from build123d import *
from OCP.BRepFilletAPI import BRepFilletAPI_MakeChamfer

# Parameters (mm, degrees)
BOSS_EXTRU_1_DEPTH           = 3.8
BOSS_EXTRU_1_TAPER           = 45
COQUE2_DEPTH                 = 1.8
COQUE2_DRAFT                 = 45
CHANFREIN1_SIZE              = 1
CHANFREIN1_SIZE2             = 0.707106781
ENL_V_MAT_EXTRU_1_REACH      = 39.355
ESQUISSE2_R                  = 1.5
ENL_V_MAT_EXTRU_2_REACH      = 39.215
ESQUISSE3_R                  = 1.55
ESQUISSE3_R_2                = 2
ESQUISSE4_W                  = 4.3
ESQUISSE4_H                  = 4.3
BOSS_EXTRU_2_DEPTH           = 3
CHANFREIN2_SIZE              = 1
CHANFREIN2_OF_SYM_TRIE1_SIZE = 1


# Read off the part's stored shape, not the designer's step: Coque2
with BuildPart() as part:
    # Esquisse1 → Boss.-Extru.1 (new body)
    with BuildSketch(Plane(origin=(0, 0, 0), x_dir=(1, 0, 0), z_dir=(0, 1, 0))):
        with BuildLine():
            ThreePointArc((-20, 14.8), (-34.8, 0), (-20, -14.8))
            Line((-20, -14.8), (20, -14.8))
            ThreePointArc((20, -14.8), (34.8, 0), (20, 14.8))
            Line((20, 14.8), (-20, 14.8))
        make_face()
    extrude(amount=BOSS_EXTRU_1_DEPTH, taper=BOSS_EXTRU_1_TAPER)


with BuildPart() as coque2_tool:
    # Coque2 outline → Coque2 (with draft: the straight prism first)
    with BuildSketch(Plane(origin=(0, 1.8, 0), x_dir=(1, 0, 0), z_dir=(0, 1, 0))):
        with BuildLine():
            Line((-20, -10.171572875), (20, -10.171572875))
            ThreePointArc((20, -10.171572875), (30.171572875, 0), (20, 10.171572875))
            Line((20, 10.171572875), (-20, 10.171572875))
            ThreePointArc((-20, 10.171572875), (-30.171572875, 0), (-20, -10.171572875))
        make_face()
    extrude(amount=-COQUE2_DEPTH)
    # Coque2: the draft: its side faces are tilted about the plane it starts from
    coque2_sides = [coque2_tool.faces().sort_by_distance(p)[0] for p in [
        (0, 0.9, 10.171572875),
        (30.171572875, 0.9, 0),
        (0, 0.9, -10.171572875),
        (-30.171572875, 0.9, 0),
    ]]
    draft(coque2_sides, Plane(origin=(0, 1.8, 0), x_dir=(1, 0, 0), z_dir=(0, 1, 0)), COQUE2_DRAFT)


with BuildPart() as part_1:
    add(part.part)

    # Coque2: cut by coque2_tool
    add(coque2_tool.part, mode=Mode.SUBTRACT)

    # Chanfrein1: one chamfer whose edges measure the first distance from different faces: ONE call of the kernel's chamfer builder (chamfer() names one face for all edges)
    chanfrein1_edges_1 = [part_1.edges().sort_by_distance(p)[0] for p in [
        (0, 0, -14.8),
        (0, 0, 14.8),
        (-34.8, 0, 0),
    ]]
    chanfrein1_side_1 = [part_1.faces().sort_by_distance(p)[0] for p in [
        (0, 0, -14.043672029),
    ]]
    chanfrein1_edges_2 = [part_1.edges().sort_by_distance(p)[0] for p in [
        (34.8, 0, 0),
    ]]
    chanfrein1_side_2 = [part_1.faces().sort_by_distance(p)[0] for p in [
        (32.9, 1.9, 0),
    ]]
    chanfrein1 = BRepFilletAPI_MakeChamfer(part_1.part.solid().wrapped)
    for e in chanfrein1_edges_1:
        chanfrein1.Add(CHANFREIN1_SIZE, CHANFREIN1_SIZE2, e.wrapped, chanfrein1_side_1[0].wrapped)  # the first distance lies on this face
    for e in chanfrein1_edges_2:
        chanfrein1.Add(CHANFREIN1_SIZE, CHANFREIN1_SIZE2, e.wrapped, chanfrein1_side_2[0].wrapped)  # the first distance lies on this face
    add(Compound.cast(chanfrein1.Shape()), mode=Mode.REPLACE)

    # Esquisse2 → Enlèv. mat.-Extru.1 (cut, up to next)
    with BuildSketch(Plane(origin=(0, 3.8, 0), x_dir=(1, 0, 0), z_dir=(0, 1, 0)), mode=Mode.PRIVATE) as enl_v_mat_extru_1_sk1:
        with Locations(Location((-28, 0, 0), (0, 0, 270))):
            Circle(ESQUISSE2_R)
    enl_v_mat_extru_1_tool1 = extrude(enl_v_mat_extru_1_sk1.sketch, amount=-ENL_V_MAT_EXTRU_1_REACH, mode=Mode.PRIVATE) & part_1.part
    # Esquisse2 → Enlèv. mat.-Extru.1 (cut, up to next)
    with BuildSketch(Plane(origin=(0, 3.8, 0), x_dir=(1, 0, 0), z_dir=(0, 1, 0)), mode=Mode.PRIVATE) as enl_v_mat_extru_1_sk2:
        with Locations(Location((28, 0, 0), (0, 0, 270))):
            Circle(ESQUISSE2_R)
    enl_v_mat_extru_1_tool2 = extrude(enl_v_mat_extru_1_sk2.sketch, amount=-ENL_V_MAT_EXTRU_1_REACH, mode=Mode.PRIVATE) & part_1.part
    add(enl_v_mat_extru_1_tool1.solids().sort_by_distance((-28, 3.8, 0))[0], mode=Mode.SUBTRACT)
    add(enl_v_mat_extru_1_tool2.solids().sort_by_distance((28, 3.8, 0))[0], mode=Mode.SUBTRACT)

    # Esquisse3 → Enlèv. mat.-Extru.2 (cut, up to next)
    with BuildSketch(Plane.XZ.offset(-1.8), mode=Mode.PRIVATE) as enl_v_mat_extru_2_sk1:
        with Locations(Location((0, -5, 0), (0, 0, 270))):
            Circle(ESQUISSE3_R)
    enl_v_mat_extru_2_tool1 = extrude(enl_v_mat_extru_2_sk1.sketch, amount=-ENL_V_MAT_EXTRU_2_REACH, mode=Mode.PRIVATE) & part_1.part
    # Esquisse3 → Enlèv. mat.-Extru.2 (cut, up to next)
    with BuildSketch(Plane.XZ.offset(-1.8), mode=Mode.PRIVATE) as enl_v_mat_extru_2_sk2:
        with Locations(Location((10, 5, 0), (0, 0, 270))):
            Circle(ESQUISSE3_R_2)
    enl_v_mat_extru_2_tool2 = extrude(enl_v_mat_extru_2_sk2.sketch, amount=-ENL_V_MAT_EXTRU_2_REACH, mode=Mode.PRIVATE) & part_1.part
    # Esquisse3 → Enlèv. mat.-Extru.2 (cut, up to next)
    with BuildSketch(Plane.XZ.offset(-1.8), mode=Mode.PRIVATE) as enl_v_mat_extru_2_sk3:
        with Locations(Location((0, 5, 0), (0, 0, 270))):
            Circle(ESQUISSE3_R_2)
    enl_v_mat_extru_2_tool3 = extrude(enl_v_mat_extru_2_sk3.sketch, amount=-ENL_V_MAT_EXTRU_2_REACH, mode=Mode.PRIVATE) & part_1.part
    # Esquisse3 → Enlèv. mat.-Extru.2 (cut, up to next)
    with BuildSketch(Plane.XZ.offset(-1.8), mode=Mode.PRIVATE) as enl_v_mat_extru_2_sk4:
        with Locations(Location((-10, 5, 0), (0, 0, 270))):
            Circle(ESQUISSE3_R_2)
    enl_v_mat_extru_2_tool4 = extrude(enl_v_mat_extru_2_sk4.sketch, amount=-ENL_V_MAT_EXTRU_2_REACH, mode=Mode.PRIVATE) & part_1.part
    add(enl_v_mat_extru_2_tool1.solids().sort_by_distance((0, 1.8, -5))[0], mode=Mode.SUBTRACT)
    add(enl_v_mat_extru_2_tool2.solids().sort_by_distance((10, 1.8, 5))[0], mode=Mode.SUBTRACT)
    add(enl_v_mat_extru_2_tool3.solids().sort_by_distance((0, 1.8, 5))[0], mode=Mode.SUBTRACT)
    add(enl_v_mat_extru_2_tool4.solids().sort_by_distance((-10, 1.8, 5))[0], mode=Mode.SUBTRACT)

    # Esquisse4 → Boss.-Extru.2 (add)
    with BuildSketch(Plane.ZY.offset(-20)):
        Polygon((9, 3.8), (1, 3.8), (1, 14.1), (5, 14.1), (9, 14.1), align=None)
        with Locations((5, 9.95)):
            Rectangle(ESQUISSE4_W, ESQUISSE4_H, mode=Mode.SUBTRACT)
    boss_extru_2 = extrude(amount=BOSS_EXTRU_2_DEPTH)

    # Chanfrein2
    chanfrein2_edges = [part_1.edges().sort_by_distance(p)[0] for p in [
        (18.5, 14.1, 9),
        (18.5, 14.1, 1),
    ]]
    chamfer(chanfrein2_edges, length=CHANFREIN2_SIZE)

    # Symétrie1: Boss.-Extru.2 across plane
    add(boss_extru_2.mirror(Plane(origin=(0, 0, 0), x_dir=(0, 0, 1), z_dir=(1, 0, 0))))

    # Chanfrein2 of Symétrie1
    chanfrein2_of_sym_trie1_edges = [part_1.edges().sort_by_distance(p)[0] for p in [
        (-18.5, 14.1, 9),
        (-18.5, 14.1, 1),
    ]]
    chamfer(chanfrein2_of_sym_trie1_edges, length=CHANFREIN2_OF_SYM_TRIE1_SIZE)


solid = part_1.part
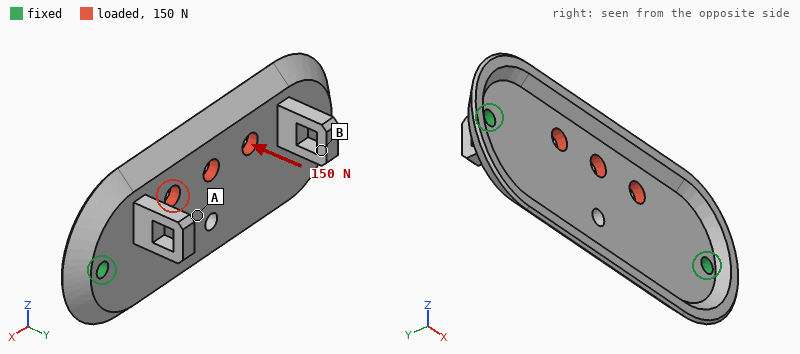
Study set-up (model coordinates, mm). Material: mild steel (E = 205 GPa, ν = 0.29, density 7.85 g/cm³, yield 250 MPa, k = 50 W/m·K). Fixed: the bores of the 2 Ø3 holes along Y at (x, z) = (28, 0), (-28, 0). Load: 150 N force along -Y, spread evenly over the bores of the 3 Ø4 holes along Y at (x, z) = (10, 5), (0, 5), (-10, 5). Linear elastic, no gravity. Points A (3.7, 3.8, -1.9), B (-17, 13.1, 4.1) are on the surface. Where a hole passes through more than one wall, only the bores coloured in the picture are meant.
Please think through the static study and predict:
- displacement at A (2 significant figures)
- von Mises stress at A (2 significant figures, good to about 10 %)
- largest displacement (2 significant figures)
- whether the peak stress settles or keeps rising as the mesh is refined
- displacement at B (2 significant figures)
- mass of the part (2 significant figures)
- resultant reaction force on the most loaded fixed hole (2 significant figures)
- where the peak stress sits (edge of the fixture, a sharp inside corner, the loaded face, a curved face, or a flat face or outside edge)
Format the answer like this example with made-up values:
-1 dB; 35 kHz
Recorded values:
21 µm; 18 MPa; 37 µm; keeps rising; 21 µm; 30 g; 110 N; edge of the fixture
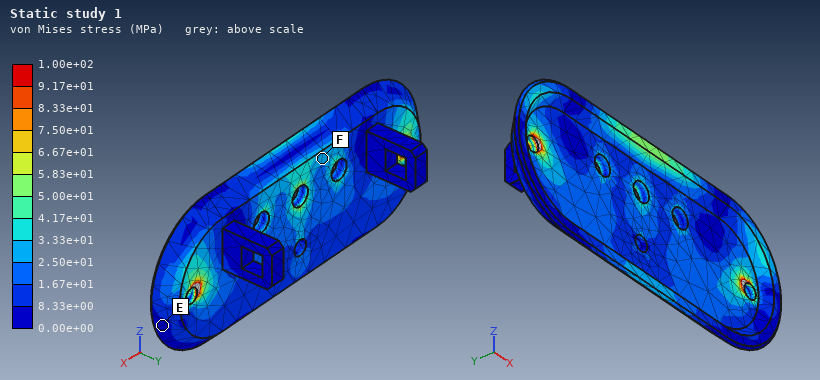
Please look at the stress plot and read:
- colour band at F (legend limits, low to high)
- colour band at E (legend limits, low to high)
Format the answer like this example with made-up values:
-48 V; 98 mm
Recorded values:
2.50e+01 to 3.33e+01 MPa; 0.00e+00 to 8.33e+00 MPa
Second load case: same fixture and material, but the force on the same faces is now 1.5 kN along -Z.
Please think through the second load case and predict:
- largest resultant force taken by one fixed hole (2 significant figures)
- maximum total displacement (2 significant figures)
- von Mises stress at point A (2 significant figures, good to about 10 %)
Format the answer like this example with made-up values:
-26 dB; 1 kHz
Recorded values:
750 N; 20 µm; 16 MPa
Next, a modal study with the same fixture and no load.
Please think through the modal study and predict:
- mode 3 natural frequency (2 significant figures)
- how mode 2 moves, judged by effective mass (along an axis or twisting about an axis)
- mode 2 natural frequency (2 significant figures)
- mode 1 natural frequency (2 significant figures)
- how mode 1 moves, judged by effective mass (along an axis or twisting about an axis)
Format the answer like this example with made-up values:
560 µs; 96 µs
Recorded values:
7800 Hz; twisting about X; 4000 Hz; 3500 Hz; along Y
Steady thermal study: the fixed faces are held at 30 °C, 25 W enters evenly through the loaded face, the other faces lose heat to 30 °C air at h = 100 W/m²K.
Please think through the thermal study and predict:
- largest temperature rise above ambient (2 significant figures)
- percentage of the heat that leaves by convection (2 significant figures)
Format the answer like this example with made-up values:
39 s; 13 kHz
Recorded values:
85 K; 58 %
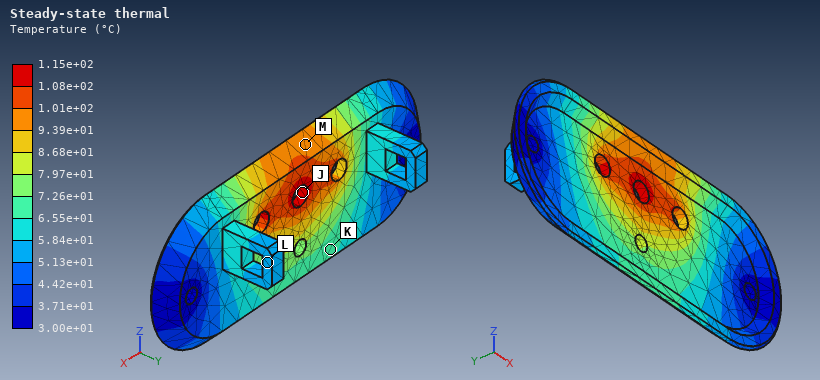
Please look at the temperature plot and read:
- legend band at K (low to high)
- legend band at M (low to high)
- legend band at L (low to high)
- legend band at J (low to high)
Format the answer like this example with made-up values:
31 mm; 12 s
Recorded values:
6.55e+01 to 7.26e+01 °C; 9.39e+01 to 1.01e+02 °C; 5.13e+01 to 5.84e+01 °C; 1.08e+02 to 1.15e+02 °C
